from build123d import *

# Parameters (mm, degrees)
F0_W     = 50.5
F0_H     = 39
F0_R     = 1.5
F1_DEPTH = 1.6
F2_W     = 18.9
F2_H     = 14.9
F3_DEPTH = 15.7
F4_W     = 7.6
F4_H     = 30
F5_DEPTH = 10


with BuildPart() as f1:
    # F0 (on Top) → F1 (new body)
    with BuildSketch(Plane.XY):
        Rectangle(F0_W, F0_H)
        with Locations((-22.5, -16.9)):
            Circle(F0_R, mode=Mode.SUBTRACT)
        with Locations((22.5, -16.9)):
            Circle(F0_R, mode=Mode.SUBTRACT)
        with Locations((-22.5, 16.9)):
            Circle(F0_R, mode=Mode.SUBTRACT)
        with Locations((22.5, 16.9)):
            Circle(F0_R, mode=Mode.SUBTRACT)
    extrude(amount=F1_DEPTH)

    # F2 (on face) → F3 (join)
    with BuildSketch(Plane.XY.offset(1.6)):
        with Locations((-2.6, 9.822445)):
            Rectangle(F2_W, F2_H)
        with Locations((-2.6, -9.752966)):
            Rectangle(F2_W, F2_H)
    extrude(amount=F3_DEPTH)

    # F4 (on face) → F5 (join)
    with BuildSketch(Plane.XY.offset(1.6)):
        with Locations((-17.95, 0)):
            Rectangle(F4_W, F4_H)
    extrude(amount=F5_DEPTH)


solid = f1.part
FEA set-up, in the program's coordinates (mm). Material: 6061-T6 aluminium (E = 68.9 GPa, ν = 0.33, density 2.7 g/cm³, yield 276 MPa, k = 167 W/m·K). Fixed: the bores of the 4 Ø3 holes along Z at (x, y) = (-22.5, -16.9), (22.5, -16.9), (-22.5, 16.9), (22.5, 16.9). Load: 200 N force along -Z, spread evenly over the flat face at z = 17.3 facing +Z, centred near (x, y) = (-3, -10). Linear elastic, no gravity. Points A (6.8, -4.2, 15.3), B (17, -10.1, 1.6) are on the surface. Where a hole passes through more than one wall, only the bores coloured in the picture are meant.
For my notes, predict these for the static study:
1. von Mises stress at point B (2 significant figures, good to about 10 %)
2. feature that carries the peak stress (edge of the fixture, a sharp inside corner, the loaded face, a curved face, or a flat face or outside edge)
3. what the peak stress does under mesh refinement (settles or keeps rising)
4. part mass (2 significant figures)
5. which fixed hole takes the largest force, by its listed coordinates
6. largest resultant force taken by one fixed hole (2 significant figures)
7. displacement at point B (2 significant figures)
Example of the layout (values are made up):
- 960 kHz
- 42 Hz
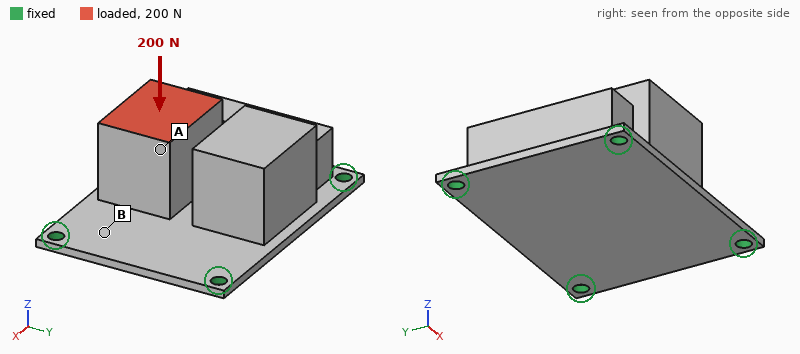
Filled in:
- 12 MPa
- edge of the fixture
- keeps rising
- 38 g
- (-22.5, -16.9)
- 120 N
- 21 µm
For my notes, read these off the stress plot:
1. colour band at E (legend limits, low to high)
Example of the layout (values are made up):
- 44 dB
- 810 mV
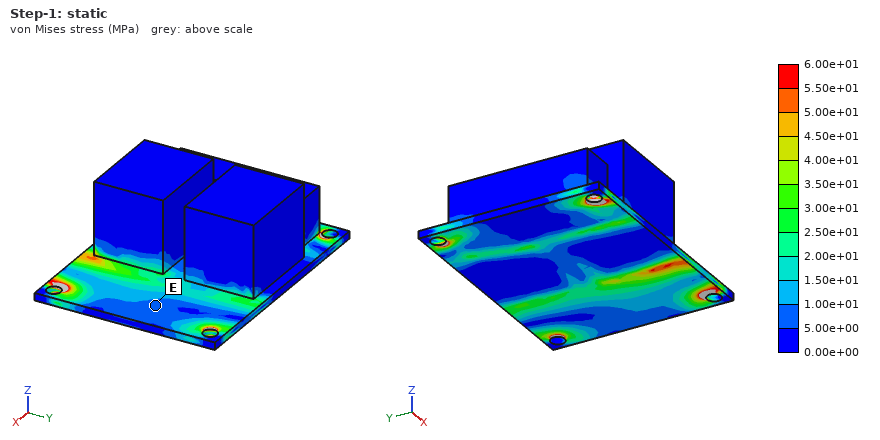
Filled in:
- 5.00e+00 to 1.00e+01 MPa
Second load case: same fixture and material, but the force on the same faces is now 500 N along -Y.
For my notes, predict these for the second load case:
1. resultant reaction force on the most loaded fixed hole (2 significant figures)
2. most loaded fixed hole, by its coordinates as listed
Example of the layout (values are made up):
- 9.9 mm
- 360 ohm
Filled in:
- 400 N
- (-22.5, 16.9)
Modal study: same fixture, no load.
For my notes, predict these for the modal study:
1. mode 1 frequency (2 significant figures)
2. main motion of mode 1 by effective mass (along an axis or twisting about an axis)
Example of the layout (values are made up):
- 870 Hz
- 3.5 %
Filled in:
- 2100 Hz
- along Z
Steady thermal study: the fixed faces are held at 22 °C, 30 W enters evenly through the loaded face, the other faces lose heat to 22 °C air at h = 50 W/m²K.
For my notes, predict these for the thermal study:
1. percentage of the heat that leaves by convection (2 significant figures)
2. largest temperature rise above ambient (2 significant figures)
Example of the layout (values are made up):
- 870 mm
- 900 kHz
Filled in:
- 20 %
- 39 K
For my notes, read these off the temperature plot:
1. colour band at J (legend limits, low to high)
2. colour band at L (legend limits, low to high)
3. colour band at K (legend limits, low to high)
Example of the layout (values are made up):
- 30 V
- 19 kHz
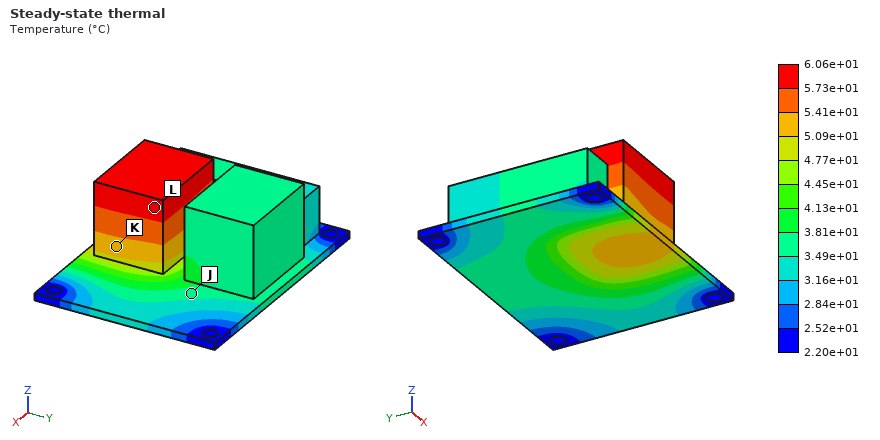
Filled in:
- 3.49e+01 to 3.81e+01 °C
- 5.73e+01 to 6.06e+01 °C
- 5.09e+01 to 5.41e+01 °C
